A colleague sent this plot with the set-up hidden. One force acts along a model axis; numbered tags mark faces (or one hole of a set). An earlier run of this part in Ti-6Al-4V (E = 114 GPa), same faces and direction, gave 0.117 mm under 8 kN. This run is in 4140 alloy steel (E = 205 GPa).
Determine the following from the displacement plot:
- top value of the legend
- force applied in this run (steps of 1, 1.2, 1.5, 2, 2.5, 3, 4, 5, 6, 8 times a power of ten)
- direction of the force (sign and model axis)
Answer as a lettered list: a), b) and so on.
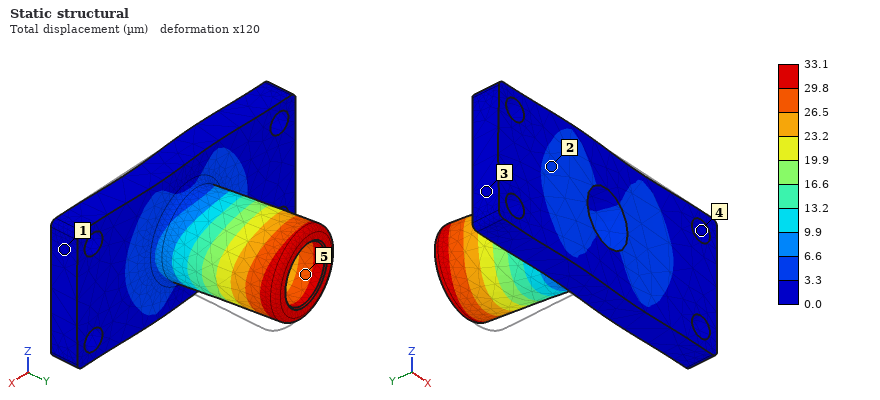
a) 33.1 µm
b) 4 kN
c) -X
